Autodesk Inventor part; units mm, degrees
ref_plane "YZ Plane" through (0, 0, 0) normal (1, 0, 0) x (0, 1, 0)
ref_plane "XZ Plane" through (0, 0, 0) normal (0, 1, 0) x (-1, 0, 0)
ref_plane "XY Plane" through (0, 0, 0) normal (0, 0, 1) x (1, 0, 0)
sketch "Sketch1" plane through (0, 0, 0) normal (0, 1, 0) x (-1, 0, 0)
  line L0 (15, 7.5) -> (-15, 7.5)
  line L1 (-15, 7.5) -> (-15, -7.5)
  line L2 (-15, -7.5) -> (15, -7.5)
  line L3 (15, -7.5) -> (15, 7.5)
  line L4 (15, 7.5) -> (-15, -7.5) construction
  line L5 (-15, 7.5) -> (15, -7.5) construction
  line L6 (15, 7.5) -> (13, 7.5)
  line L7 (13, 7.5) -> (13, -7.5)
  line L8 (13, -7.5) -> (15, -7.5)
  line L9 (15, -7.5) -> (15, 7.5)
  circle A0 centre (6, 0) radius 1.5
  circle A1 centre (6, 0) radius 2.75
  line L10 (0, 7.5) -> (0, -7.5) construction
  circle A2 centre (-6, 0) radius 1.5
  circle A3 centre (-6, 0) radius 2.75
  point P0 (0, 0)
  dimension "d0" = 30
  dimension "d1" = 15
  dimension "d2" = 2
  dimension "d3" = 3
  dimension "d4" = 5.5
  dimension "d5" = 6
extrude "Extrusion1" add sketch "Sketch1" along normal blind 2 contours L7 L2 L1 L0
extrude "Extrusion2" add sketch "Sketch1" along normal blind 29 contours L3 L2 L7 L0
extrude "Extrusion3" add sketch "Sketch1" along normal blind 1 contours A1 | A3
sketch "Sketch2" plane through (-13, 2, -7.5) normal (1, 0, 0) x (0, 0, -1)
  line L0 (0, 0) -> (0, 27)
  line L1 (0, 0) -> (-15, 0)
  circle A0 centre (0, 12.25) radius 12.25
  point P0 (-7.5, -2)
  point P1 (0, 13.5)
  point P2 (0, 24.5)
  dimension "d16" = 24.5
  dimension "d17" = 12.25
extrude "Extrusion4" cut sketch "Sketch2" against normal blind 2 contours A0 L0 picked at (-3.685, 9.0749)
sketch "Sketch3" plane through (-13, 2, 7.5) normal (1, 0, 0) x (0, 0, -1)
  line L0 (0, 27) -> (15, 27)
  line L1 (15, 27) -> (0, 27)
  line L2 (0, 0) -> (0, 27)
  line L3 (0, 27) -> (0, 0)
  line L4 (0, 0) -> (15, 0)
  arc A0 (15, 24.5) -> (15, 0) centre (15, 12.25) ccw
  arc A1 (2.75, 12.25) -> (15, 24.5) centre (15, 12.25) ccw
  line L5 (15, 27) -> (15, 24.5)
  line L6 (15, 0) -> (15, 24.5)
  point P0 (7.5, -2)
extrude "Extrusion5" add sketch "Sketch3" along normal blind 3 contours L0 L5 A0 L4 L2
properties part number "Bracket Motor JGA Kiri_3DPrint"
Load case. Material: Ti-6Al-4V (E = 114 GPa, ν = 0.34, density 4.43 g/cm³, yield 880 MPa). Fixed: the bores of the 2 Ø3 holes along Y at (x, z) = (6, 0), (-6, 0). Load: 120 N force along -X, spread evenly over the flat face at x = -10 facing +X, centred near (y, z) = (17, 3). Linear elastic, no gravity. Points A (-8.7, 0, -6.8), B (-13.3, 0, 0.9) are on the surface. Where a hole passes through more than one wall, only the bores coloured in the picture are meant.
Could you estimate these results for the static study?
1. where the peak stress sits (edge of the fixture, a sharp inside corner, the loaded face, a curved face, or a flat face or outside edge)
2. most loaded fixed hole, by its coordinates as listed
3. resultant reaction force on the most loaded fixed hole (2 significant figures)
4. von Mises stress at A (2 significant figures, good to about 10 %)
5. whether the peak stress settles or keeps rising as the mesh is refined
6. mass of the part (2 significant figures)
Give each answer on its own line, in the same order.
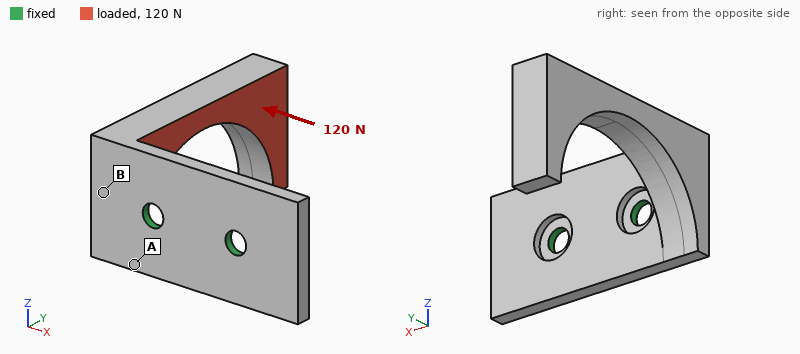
edge of the fixture
(6, 0)
340 N
160 MPa
keeps rising
7.5 g
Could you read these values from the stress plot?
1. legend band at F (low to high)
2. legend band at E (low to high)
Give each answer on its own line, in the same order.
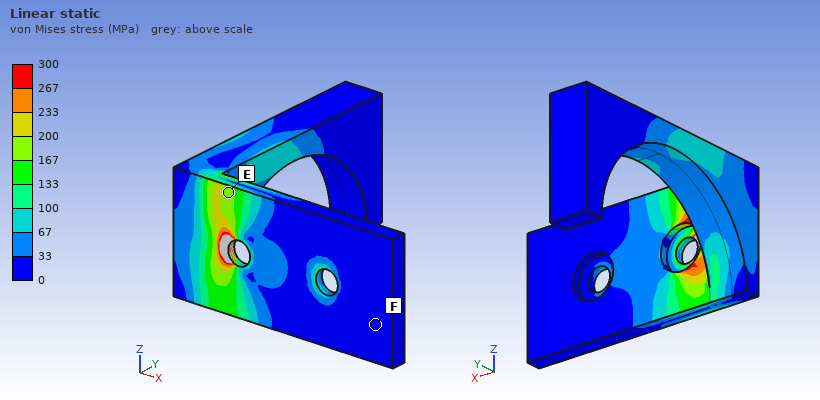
0 to 33 MPa
167 to 200 MPa
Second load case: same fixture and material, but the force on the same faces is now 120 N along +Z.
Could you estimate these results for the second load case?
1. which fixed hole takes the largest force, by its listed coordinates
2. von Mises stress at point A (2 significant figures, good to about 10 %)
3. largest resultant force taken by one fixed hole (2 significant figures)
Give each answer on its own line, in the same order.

(-6, 0)
42 MPa
120 N
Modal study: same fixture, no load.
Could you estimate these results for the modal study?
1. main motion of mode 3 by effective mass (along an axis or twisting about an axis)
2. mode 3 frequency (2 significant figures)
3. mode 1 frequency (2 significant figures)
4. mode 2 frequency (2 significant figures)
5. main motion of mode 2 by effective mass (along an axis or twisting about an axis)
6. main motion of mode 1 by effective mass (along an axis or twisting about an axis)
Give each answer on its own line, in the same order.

along Y
6000 Hz
1500 Hz
1700 Hz
along Z
along X
